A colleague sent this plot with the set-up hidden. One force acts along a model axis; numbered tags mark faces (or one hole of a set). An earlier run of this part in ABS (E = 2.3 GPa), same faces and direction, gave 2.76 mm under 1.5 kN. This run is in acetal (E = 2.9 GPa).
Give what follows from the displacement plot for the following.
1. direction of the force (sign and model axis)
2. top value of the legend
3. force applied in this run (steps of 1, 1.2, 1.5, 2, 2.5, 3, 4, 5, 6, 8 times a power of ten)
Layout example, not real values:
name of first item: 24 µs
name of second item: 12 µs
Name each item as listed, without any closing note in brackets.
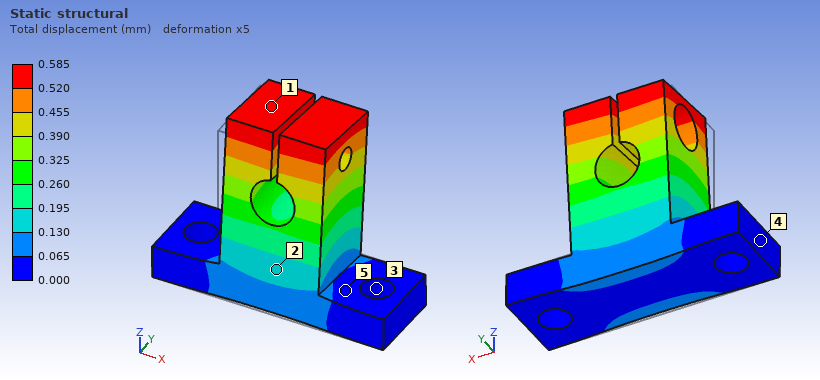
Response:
direction of the force: +Y
top value of the legend: 0.585 mm
force applied in this run: 400 N
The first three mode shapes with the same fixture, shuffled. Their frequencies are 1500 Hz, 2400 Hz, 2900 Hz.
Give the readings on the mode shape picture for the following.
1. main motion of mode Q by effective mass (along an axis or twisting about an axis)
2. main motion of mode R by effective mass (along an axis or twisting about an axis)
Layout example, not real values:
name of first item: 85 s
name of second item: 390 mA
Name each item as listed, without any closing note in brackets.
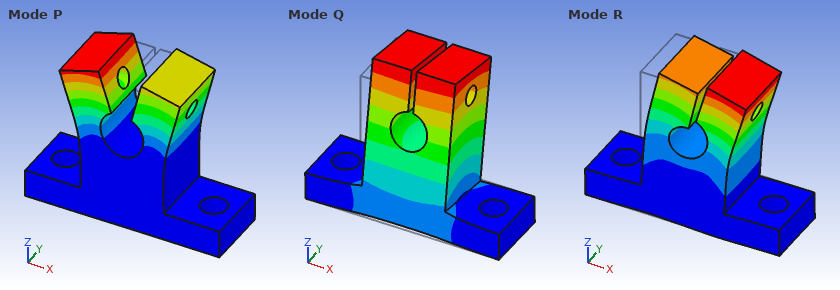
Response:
main motion of mode Q by effective mass: along Y
main motion of mode R by effective mass: along X
